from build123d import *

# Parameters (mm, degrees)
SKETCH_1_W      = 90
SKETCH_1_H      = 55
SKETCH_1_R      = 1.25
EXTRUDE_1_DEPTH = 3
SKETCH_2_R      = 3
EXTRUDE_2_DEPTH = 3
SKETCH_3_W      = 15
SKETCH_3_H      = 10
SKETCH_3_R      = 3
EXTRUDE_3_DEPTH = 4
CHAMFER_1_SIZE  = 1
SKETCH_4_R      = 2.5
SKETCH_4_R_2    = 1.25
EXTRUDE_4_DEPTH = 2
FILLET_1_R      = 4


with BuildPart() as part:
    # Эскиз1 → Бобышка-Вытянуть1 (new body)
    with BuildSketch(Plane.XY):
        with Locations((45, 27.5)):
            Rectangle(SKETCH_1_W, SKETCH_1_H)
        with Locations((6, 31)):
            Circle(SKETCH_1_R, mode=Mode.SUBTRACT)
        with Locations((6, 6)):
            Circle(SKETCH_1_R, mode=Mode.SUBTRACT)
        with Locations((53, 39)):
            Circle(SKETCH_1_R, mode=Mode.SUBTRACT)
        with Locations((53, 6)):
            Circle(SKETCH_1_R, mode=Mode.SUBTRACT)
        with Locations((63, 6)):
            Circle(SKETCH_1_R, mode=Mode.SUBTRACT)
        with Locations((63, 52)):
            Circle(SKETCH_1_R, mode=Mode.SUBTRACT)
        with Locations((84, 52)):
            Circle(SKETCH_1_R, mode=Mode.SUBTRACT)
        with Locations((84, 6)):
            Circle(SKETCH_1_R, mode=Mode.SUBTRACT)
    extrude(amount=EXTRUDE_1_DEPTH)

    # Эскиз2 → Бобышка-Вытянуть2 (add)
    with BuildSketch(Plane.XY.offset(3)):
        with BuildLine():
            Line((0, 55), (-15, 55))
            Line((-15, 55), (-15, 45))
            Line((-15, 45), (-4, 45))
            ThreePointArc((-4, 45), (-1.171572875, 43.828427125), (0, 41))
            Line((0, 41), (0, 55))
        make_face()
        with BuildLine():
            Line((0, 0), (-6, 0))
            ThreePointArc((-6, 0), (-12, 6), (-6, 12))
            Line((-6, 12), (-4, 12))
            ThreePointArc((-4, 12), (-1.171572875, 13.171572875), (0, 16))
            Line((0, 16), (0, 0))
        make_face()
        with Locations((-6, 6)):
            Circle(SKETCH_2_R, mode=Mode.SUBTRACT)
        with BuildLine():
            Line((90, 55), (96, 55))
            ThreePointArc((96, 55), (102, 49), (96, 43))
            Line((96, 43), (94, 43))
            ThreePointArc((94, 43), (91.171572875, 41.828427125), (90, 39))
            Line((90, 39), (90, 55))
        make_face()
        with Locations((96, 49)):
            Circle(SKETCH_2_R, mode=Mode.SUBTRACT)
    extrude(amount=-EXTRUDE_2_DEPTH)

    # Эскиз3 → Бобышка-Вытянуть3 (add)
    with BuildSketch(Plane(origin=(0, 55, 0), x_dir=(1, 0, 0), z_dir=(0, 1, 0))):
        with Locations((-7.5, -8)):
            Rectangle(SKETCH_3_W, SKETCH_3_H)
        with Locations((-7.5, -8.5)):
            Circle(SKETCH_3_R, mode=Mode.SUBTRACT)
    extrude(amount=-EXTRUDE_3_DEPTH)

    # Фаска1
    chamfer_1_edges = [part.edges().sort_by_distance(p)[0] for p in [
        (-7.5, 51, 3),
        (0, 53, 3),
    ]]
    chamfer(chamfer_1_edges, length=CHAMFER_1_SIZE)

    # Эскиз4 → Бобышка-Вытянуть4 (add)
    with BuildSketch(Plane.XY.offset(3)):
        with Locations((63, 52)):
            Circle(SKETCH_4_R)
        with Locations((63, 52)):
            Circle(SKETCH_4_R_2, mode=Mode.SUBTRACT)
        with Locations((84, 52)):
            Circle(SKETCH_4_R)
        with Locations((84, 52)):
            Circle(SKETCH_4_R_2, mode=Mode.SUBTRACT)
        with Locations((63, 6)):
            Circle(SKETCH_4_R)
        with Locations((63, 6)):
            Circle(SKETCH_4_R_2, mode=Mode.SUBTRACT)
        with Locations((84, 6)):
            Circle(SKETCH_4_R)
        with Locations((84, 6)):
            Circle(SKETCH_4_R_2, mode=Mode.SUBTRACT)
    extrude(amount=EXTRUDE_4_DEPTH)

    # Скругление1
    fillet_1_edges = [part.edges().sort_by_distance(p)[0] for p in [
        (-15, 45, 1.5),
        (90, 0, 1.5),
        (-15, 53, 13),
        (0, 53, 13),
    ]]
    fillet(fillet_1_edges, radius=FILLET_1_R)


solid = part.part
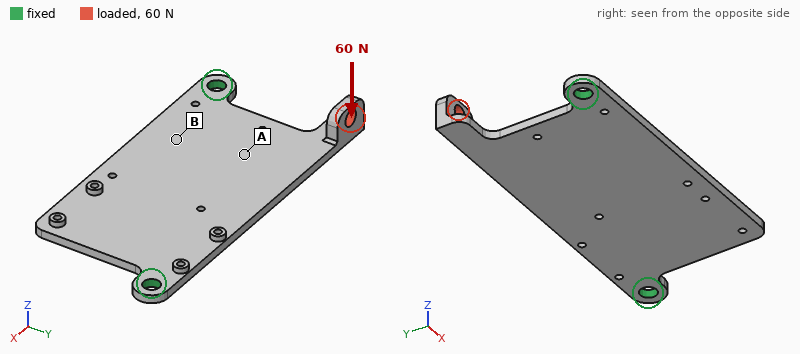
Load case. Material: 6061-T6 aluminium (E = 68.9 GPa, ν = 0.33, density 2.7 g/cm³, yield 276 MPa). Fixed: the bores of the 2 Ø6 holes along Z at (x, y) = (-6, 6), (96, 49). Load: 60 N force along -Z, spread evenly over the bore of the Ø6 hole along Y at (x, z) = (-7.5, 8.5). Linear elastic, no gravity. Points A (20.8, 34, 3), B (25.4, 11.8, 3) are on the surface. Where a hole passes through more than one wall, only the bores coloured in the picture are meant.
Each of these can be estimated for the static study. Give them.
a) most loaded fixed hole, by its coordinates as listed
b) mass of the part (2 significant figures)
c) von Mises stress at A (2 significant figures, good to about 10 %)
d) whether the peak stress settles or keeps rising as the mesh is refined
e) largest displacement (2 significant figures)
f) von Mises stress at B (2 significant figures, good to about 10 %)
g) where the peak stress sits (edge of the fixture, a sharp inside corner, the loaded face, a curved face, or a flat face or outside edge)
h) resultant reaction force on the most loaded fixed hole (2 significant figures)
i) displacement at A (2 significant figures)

(-6, 6)
44 g
24 MPa
keeps rising
0.77 mm
9.2 MPa
edge of the fixture
57 N
0.18 mm
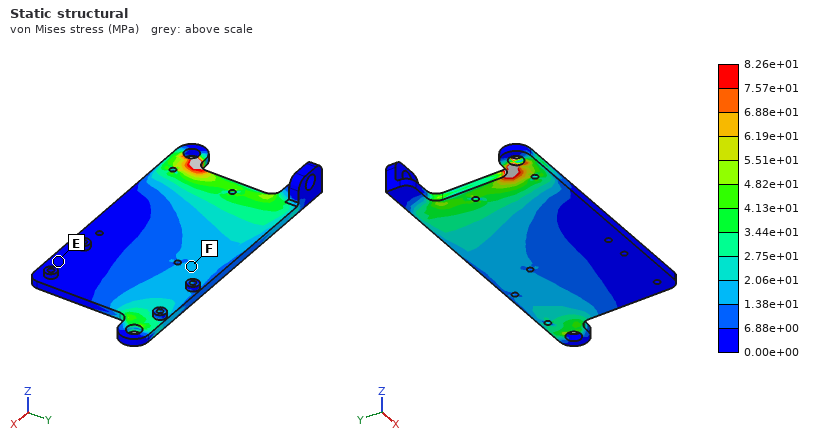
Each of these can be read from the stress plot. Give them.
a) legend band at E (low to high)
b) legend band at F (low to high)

0.00e+00 to 6.88e+00 MPa
1.38e+01 to 2.06e+01 MPa
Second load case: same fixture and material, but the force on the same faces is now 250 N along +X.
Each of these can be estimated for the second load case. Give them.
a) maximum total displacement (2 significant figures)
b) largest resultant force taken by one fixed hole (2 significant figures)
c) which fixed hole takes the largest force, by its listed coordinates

0.47 mm
160 N
(96, 49)
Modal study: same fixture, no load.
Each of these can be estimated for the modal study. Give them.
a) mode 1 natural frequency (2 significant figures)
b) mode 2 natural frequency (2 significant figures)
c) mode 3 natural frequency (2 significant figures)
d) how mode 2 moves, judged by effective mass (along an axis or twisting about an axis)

660 Hz
880 Hz
1600 Hz
along Z
